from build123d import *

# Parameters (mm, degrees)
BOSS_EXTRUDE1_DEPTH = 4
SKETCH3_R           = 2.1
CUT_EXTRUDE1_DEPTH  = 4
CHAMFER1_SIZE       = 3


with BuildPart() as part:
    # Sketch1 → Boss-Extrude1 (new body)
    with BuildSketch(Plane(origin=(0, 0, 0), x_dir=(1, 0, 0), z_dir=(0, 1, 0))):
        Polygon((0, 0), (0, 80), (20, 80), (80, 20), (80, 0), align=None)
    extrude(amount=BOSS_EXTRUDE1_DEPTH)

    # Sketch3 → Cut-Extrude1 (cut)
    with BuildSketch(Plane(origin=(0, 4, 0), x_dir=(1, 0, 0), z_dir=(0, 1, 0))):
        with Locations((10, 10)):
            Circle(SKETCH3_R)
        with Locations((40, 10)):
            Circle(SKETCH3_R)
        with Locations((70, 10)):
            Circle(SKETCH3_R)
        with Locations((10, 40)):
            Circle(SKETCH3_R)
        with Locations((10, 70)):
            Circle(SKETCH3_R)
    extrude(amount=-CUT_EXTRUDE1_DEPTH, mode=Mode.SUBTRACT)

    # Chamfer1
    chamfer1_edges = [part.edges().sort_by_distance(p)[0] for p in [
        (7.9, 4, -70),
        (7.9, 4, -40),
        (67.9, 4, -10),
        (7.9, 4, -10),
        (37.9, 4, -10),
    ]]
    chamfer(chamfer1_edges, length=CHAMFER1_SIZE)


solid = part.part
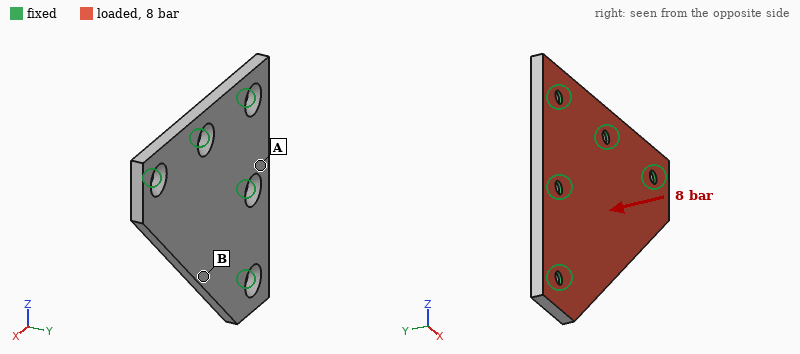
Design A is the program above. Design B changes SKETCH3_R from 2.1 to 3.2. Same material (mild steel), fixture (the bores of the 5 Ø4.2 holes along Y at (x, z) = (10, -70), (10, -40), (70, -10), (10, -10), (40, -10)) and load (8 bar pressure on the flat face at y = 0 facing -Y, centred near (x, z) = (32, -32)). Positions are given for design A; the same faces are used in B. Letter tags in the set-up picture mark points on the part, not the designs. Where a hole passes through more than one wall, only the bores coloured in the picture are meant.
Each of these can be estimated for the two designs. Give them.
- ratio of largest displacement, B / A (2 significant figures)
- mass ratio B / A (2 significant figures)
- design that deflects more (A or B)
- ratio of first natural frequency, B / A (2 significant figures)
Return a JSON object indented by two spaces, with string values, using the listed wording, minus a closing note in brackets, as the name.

{
  "ratio of largest displacement, B / A": "0.81",
  "mass ratio B / A": "0.97",
  "design that deflects more": "A",
  "ratio of first natural frequency, B / A": "1.1"
}
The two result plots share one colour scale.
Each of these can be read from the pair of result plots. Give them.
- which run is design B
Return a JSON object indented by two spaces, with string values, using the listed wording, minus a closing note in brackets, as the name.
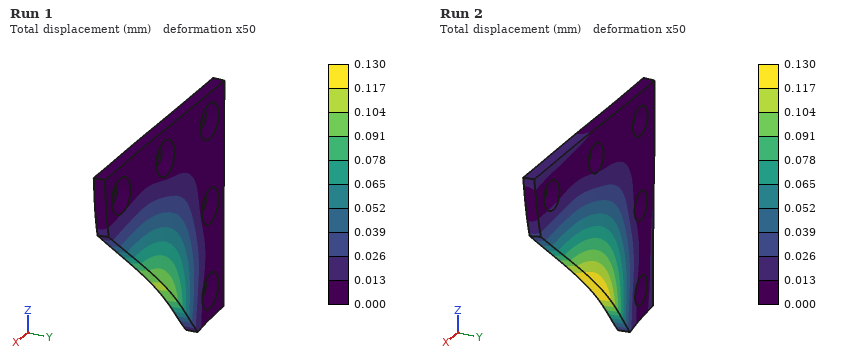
{
  "which run is design B": "Run 1"
}
